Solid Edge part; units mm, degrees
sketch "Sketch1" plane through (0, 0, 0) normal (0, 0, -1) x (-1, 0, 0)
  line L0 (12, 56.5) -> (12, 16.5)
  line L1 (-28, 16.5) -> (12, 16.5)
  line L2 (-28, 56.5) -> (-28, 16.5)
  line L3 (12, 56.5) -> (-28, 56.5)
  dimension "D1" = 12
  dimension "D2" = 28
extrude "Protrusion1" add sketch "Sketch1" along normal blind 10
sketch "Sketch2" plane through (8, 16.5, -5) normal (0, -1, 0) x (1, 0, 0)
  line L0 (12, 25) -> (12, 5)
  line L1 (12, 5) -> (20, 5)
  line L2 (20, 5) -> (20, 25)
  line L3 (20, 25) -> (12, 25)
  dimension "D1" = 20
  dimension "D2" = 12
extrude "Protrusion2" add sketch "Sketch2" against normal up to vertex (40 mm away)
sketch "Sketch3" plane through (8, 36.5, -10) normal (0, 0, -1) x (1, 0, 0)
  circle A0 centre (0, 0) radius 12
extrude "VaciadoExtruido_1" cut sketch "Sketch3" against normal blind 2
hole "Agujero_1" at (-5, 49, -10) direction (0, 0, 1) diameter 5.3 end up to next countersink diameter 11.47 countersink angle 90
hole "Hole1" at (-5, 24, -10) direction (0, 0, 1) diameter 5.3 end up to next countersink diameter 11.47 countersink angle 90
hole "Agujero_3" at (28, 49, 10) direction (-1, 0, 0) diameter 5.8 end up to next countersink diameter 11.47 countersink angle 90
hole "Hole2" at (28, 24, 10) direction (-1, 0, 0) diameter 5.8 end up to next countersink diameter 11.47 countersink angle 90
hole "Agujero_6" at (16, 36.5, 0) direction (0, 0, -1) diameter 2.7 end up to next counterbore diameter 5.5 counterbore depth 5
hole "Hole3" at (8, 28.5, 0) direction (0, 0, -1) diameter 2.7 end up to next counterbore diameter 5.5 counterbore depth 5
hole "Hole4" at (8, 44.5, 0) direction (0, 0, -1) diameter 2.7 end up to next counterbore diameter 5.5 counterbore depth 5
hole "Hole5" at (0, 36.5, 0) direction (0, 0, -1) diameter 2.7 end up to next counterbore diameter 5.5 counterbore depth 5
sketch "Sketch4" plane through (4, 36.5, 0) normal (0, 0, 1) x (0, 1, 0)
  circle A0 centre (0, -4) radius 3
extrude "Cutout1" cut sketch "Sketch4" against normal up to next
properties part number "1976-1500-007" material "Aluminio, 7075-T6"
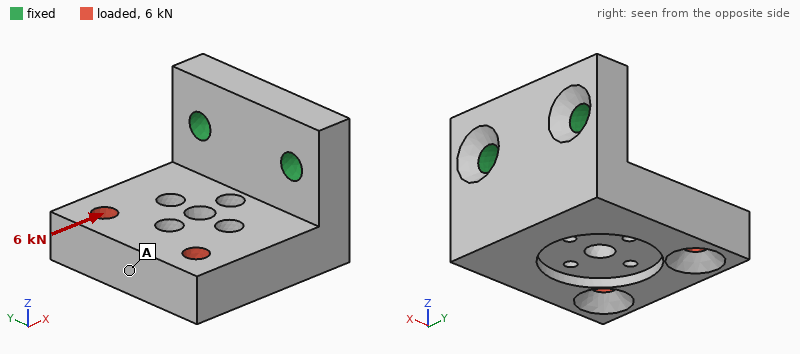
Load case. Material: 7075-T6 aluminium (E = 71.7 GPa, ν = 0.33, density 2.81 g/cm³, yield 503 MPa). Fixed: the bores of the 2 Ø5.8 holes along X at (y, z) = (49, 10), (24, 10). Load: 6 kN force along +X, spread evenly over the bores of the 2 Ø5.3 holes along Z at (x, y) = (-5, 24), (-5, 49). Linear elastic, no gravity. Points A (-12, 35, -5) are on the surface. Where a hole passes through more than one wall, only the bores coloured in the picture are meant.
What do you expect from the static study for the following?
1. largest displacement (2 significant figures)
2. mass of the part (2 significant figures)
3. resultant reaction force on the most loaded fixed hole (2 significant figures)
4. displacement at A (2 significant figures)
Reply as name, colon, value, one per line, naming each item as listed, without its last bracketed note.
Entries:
largest displacement: 0.24 mm
mass of the part: 55 g
resultant reaction force on the most loaded fixed hole: 3.0 kN
displacement at A: 0.23 mm
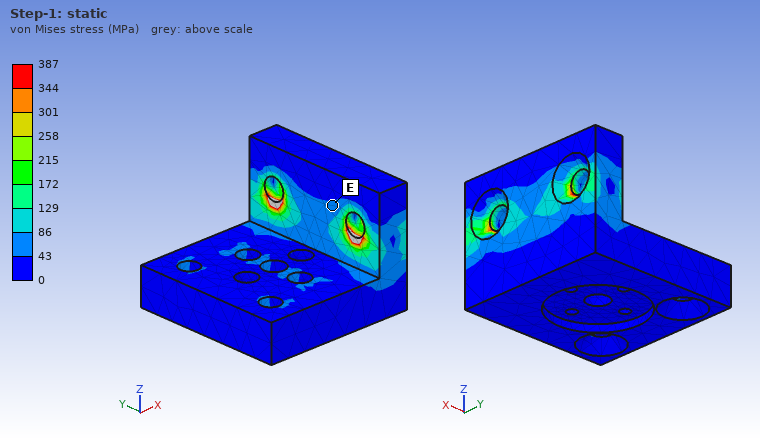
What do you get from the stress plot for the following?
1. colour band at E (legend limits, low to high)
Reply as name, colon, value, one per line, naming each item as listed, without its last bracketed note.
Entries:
colour band at E: 43 to 86 MPa
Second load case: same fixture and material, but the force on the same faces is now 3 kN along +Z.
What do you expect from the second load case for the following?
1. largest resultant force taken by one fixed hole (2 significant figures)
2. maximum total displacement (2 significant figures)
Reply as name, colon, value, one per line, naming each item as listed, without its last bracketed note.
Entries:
largest resultant force taken by one fixed hole: 1.6 kN
maximum total displacement: 0.62 mm
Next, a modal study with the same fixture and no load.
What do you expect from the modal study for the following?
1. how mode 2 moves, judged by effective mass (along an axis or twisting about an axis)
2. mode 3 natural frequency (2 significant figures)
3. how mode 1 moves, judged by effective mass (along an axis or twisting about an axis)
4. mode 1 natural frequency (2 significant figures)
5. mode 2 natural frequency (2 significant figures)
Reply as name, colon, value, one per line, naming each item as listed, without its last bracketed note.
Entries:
how mode 2 moves, judged by effective mass: along Y
mode 3 natural frequency: 9500 Hz
how mode 1 moves, judged by effective mass: along Z
mode 1 natural frequency: 2900 Hz
mode 2 natural frequency: 5700 Hz
